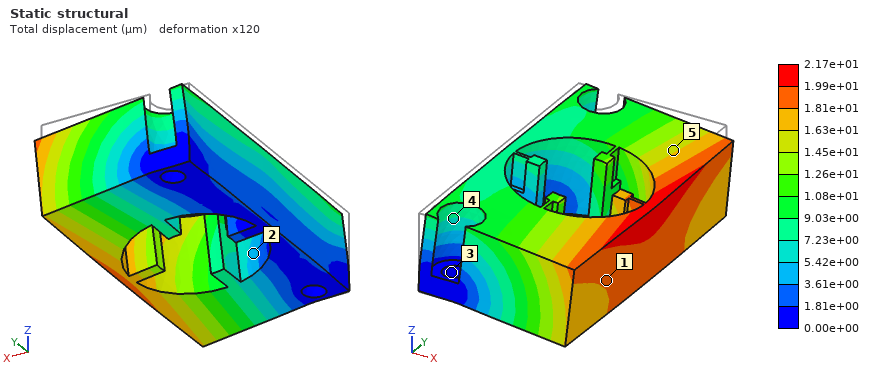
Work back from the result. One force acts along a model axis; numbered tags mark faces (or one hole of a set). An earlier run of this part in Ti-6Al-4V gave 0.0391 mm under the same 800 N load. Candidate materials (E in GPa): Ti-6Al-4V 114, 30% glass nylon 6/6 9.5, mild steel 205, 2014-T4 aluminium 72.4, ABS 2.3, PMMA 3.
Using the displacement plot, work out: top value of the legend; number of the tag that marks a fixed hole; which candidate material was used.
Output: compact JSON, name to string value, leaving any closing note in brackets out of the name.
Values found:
{"top value of the legend": "2.17e+01 µm", "number of the tag that marks a fixed hole": "3", "which candidate material was used": "mild steel"}
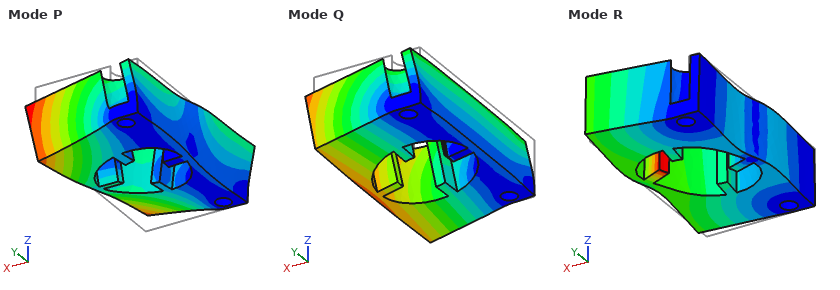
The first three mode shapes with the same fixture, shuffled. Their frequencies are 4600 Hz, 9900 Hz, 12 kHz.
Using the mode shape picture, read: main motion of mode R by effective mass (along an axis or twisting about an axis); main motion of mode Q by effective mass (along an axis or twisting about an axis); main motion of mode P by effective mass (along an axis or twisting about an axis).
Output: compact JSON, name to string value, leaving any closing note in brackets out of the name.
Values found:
{"main motion of mode R by effective mass": "along Y", "main motion of mode Q by effective mass": "along Z", "main motion of mode P by effective mass": "twisting about X"}
